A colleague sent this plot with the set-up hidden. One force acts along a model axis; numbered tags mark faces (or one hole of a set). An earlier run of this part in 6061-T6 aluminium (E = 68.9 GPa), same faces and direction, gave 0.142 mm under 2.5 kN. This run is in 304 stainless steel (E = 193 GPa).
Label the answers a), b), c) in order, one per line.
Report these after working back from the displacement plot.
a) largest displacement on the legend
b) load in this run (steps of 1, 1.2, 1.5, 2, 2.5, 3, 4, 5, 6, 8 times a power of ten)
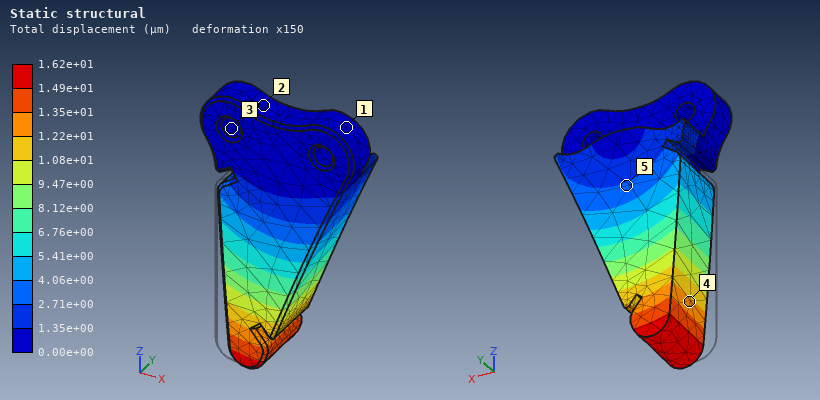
a) 1.62e+01 µm
b) 800 N
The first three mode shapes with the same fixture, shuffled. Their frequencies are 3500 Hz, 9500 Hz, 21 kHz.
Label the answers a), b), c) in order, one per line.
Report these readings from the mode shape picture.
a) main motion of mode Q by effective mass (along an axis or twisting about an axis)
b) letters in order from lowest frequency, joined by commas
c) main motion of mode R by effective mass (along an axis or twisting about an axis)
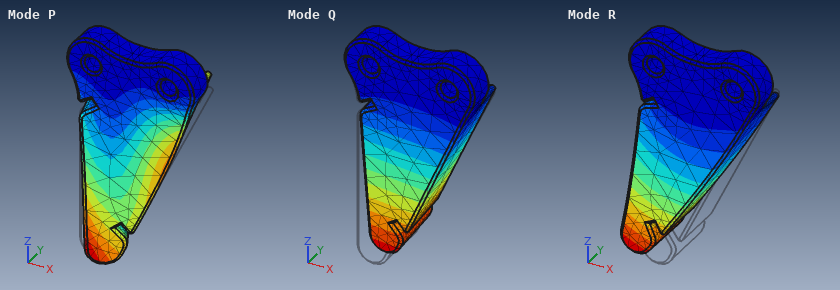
a) along Y
b) Q, R, P
c) along X
